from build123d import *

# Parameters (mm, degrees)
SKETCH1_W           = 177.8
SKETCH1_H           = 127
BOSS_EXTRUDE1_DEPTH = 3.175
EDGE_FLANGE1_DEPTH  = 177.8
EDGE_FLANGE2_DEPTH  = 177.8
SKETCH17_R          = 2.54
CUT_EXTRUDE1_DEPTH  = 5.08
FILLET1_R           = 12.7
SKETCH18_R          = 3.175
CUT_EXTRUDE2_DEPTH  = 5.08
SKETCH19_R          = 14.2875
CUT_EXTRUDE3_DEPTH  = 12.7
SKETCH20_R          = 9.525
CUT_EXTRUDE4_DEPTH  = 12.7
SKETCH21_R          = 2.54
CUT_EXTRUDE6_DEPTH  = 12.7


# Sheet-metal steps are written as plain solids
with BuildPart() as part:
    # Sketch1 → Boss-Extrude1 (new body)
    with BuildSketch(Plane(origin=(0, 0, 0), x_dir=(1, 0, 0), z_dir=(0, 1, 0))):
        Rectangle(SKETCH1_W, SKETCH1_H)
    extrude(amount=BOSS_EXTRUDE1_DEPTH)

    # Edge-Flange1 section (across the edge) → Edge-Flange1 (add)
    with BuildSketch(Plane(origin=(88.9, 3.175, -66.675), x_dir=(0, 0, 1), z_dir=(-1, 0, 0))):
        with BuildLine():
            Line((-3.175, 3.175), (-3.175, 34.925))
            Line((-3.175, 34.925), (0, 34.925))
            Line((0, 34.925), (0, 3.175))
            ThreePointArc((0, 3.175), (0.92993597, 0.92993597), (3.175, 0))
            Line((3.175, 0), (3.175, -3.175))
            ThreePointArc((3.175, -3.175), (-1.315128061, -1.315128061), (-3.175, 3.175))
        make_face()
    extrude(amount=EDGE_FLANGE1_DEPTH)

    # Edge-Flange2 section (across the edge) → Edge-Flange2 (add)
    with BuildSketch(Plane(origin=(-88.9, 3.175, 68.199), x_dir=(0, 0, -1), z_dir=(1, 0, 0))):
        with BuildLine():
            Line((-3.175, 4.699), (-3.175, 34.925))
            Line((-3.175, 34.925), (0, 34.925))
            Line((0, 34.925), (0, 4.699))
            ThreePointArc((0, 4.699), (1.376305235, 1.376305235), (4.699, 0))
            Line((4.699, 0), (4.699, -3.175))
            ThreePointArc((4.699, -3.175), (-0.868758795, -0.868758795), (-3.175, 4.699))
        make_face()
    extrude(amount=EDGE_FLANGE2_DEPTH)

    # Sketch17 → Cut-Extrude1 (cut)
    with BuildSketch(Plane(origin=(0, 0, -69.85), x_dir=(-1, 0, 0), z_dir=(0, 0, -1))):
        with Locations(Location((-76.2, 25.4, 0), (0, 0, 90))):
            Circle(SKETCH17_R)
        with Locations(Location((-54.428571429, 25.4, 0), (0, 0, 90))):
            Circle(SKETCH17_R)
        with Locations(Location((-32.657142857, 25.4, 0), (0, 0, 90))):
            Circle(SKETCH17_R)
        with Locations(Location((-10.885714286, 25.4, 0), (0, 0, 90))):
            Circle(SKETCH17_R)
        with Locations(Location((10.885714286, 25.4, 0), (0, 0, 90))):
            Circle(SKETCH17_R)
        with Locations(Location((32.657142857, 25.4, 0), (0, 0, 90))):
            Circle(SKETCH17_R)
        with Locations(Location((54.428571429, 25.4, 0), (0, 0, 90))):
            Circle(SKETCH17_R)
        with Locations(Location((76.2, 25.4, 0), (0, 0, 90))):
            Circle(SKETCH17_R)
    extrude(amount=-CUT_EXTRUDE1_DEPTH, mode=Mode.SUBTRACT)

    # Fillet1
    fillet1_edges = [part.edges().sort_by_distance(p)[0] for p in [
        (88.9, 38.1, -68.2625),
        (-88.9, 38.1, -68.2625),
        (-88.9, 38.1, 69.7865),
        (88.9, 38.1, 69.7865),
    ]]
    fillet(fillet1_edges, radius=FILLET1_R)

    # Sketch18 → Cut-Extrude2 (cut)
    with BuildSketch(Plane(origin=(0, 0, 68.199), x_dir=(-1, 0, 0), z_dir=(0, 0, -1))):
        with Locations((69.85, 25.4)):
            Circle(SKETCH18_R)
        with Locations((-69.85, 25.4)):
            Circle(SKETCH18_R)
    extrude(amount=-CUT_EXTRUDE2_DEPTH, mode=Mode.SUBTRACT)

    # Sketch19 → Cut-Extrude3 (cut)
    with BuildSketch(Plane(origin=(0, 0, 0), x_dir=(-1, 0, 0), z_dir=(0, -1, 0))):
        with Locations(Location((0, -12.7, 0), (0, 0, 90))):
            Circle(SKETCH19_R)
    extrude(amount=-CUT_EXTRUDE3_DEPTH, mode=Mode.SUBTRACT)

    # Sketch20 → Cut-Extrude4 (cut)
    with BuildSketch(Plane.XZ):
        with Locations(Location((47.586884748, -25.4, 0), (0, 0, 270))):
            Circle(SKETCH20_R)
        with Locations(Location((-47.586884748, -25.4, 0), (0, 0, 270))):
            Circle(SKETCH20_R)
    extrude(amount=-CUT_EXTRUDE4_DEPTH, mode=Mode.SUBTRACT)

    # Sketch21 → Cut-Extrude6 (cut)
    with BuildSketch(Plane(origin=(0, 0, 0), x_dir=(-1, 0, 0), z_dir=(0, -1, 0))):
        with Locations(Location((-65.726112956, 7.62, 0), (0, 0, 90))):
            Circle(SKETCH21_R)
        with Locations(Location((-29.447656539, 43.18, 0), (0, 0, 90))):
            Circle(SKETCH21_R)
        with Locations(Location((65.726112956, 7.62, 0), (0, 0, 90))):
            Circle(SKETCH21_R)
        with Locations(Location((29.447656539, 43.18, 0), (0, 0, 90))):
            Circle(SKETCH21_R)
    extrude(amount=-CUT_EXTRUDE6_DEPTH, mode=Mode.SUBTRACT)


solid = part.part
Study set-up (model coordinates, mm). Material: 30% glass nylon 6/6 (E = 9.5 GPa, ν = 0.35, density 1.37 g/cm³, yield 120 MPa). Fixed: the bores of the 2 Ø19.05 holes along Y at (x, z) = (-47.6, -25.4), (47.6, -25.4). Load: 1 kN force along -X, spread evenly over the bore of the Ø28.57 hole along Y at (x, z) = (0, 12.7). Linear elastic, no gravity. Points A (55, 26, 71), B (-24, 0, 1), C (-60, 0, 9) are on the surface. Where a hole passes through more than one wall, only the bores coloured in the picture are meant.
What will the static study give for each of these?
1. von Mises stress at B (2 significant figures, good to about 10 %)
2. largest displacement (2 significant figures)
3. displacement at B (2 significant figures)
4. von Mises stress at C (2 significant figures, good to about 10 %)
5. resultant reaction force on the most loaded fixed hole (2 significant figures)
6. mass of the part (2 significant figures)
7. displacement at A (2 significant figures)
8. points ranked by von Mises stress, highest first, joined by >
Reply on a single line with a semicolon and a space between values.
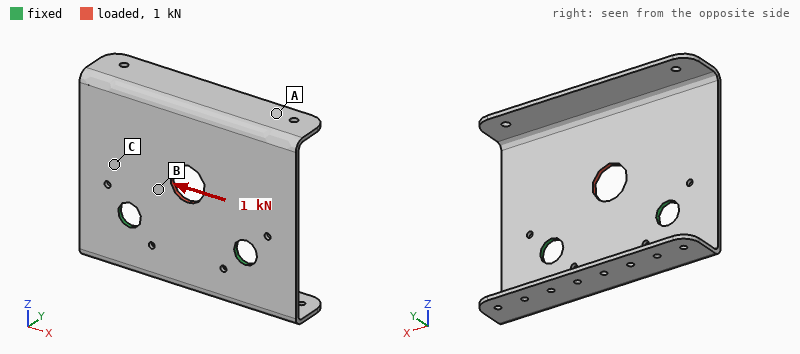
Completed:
4.2 MPa; 45 µm; 19 µm; 1.7 MPa; 600 N; 150 g; 40 µm; B > C > A
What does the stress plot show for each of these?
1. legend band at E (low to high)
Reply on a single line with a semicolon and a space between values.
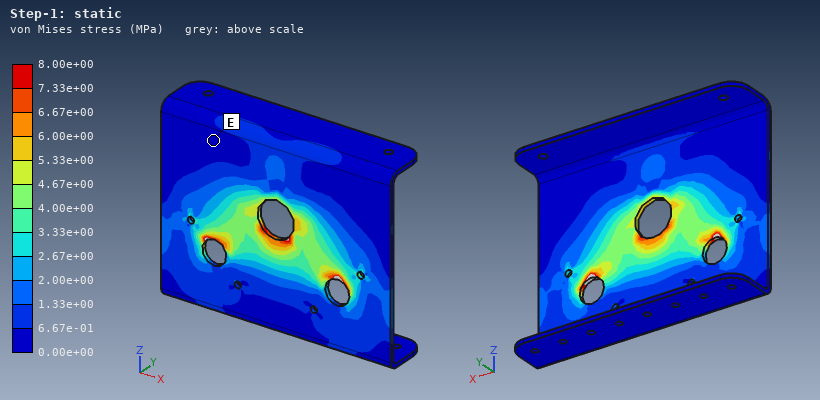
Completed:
0.00e+00 to 6.67e-01 MPa
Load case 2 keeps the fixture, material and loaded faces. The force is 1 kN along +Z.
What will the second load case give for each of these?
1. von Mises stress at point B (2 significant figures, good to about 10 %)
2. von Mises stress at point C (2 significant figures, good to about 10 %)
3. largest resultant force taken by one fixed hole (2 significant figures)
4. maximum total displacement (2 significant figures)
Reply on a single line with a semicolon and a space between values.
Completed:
3.3 MPa; 0.95 MPa; 520 N; 28 µm
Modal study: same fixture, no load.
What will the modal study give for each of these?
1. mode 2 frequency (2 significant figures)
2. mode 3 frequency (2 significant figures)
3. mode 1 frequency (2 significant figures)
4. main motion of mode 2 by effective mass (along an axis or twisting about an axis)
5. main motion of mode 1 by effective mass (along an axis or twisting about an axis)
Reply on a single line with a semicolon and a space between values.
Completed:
170 Hz; 340 Hz; 99 Hz; twisting about Z; along Y
